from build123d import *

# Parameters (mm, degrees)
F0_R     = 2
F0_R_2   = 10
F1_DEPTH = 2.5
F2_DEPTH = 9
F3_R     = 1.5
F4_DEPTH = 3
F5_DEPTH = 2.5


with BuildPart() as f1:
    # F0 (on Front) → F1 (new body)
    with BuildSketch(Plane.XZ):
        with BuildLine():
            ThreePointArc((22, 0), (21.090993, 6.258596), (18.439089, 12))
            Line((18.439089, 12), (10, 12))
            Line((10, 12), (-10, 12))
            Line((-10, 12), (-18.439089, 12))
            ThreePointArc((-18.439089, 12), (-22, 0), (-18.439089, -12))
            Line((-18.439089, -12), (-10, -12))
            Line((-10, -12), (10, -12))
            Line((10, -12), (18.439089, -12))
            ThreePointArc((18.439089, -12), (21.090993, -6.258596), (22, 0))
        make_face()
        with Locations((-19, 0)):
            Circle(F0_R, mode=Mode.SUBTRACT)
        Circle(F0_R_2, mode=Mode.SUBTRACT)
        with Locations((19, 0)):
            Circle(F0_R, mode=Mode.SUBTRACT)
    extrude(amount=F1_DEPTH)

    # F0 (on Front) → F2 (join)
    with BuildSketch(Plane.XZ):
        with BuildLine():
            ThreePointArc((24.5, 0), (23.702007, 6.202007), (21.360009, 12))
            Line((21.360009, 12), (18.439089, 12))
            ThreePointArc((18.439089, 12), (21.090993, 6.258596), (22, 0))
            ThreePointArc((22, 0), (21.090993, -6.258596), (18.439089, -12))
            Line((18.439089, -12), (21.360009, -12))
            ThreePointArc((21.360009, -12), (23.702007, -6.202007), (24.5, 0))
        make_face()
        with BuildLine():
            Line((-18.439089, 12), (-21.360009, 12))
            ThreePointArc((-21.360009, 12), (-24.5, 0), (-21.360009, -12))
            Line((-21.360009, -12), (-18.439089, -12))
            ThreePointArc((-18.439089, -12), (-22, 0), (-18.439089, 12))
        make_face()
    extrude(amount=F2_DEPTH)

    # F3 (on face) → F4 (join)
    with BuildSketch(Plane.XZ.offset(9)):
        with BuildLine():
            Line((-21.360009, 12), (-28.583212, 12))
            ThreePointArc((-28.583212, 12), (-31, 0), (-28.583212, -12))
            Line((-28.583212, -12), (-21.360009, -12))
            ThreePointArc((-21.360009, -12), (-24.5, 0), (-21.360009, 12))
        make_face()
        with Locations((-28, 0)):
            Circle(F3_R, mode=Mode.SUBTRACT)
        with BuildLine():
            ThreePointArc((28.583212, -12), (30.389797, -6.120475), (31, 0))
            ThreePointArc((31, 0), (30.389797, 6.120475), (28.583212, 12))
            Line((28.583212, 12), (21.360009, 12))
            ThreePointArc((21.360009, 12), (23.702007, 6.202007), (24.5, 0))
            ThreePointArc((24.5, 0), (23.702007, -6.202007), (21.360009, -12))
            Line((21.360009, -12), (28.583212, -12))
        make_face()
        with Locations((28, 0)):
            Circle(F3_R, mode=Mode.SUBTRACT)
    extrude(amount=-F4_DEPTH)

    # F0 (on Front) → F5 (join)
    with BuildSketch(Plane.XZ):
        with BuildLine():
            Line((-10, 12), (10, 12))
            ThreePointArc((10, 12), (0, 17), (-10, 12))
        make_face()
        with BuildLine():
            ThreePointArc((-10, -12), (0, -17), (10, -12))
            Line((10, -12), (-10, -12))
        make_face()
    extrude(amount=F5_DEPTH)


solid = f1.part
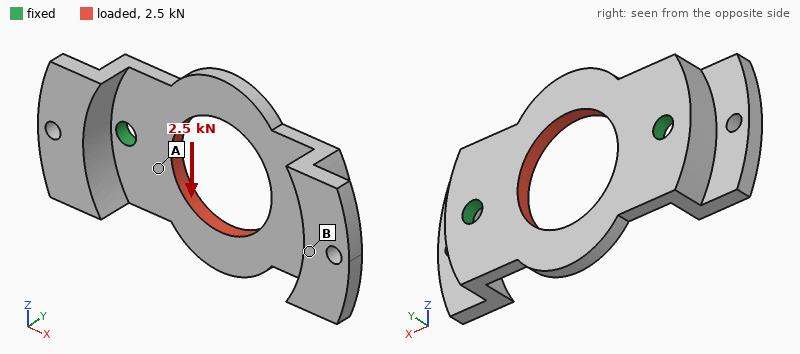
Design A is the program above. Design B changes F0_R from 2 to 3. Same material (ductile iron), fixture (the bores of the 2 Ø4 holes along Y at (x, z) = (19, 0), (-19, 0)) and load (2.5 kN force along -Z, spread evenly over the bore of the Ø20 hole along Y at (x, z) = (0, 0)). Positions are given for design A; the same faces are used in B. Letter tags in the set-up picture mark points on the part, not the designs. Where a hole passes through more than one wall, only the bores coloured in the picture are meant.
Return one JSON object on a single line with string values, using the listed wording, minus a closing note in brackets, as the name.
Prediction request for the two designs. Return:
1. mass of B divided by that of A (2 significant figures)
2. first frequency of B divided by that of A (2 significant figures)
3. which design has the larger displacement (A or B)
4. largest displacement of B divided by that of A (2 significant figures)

{"mass of B divided by that of A": "0.98", "first frequency of B divided by that of A": "1.1", "which design has the larger displacement": "A", "largest displacement of B divided by that of A": "0.90"}
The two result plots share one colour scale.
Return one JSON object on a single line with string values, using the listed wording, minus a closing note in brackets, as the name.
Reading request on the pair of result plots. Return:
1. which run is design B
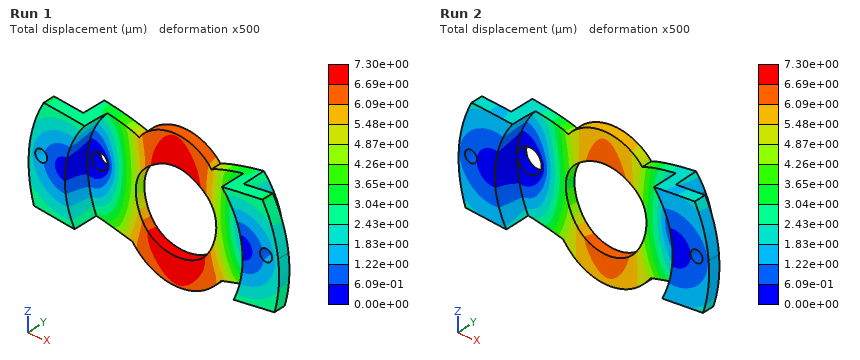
{"which run is design B": "Run 2"}
